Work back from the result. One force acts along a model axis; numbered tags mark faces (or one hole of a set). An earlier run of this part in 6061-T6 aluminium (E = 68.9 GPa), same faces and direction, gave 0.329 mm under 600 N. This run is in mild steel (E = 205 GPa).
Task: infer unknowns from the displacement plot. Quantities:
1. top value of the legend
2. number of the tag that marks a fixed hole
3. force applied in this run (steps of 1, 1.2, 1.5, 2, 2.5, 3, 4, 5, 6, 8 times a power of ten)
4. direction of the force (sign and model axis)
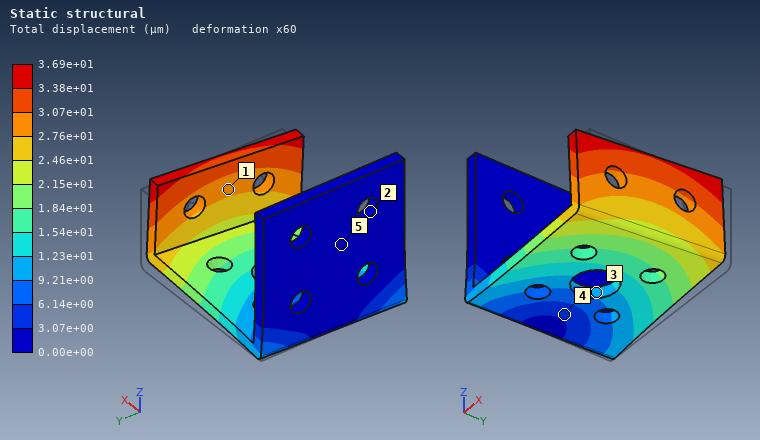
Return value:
3.69e+01 µm
2
200 N
-Y
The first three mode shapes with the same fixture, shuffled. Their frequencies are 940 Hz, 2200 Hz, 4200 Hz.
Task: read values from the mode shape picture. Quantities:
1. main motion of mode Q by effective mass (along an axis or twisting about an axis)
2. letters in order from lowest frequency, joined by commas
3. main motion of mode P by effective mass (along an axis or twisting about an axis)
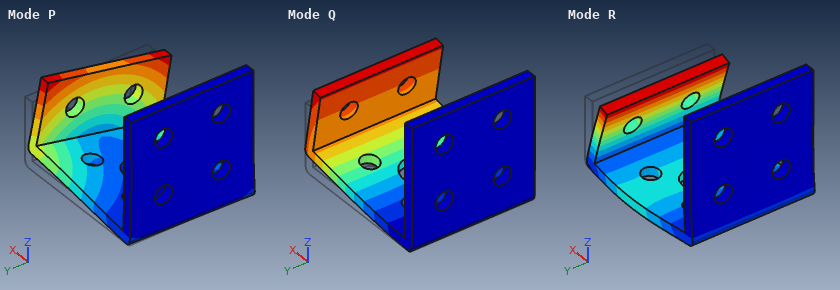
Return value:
along Z
Q, P, R
along Y
